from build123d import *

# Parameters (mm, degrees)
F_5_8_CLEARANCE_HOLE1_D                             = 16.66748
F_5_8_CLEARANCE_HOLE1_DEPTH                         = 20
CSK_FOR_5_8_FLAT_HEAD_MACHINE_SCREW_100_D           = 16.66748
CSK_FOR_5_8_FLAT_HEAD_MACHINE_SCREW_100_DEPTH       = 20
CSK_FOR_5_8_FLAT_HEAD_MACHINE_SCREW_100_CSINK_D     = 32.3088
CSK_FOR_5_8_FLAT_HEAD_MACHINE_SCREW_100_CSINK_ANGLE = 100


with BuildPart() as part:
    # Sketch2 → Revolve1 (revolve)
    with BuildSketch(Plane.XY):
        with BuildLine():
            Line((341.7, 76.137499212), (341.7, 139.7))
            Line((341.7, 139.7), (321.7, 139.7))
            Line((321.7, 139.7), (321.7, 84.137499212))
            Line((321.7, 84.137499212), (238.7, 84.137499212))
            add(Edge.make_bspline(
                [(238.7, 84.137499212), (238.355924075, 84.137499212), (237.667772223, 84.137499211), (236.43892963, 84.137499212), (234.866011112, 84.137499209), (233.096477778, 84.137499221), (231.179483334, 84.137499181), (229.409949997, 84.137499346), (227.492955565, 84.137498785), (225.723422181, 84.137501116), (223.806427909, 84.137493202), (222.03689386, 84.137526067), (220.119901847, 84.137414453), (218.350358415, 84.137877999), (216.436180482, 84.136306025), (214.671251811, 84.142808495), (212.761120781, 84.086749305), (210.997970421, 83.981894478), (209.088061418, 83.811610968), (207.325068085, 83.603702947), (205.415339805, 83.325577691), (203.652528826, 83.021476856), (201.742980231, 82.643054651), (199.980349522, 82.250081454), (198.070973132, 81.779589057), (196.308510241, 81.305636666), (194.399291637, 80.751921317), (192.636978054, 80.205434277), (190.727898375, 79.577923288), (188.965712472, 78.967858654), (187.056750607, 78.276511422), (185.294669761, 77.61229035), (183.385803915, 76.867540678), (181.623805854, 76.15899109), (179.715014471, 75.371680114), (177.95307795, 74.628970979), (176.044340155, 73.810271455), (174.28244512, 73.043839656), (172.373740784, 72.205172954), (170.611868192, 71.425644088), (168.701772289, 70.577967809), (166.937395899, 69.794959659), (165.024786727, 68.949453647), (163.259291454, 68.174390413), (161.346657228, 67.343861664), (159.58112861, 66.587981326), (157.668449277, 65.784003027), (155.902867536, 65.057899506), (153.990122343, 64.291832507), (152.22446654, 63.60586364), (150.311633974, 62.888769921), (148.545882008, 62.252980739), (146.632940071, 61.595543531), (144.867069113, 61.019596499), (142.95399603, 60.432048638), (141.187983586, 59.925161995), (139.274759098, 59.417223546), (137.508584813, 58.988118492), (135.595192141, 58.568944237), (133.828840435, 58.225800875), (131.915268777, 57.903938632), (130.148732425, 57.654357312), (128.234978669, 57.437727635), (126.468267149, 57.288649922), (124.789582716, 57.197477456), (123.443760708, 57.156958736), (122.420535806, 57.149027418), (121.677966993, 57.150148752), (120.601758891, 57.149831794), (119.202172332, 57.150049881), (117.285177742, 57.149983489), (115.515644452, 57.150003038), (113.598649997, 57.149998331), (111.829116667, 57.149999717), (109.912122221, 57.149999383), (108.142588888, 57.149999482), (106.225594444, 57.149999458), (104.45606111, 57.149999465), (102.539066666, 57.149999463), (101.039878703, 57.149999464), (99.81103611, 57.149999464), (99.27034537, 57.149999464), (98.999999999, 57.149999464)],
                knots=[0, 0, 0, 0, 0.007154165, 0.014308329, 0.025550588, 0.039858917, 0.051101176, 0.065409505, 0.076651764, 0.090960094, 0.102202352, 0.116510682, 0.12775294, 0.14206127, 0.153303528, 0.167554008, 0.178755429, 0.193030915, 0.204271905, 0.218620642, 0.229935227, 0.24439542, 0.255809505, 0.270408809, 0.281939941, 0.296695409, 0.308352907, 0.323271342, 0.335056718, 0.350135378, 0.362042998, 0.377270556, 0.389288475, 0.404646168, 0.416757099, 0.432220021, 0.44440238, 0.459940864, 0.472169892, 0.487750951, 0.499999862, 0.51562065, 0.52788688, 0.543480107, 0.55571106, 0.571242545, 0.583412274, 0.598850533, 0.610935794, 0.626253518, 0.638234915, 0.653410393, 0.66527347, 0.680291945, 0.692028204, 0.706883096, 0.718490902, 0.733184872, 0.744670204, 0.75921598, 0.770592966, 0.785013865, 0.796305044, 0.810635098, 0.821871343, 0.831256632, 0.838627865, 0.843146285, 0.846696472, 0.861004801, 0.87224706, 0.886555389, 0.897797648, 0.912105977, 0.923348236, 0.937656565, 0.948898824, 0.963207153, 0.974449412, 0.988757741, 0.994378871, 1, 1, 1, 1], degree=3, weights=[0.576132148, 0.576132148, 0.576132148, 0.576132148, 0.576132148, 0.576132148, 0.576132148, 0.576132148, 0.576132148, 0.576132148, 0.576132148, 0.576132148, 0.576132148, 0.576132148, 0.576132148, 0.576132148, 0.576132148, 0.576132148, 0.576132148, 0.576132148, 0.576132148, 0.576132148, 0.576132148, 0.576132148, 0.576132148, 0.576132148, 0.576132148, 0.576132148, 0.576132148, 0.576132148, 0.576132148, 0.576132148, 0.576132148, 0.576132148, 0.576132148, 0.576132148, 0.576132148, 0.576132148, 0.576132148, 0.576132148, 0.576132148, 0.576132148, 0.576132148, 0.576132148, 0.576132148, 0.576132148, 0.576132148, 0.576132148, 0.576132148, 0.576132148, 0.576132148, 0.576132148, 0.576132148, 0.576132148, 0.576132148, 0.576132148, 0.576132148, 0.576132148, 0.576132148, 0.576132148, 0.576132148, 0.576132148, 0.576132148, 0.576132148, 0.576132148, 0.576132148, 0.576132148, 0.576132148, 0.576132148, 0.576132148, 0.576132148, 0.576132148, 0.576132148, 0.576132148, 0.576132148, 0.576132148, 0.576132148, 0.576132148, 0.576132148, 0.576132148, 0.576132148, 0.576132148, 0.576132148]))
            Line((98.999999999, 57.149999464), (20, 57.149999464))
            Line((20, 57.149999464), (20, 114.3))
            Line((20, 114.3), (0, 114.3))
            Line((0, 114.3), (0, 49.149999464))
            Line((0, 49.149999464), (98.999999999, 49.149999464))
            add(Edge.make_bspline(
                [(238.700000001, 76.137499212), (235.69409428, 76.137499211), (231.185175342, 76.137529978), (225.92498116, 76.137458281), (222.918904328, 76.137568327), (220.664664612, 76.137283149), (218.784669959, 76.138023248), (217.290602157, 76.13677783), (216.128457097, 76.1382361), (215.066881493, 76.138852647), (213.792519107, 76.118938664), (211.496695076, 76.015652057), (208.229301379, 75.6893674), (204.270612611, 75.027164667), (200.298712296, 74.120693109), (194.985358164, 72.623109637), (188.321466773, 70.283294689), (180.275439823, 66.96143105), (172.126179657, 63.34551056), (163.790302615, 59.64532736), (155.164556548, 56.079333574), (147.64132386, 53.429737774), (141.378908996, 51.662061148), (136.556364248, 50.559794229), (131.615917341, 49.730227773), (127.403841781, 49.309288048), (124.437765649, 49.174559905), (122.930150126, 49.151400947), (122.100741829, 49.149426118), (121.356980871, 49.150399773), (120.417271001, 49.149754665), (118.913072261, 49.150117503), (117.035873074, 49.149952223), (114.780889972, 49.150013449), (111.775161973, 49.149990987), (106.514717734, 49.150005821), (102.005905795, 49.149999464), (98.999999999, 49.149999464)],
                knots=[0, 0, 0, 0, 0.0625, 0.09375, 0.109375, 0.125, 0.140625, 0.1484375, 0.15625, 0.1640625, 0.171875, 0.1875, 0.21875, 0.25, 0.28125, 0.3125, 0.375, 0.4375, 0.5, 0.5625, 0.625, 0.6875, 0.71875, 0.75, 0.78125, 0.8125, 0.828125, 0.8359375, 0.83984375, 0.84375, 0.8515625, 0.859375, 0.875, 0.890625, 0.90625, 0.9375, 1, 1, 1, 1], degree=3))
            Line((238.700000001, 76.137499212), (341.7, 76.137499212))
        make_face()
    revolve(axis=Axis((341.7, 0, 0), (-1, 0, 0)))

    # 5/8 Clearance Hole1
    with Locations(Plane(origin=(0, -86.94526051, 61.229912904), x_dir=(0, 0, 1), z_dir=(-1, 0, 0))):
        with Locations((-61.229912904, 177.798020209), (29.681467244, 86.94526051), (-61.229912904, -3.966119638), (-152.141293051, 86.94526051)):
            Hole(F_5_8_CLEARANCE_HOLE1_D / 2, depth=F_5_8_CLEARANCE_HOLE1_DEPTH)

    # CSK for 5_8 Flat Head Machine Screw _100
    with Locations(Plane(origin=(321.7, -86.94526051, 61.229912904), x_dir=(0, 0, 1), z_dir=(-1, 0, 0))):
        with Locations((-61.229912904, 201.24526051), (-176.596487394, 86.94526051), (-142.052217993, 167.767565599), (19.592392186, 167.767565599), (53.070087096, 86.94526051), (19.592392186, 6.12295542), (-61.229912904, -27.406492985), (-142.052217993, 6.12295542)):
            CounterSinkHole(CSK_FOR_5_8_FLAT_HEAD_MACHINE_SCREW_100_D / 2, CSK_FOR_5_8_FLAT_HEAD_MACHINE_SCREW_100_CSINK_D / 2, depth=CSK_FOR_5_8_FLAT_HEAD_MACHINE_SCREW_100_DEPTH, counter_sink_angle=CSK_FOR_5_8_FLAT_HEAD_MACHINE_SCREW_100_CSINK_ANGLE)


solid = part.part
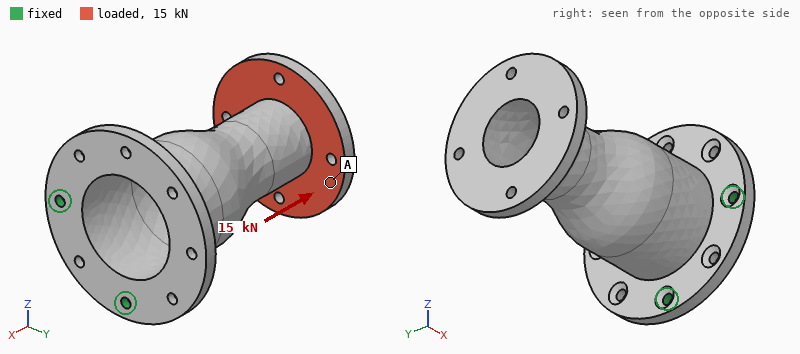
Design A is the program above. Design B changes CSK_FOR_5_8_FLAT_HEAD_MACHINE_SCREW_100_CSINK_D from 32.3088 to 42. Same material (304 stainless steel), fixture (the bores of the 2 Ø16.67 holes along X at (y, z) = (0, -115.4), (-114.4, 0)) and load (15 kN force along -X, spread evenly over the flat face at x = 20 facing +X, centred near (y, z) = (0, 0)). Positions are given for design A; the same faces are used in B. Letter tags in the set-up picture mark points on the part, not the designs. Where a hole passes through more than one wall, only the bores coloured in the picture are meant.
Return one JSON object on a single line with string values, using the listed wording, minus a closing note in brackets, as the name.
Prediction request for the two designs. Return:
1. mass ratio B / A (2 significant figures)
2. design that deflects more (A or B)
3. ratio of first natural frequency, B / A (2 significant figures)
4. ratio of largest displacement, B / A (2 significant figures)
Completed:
{"mass ratio B / A": "0.99", "design that deflects more": "B", "ratio of first natural frequency, B / A": "0.86", "ratio of largest displacement, B / A": "1.4"}
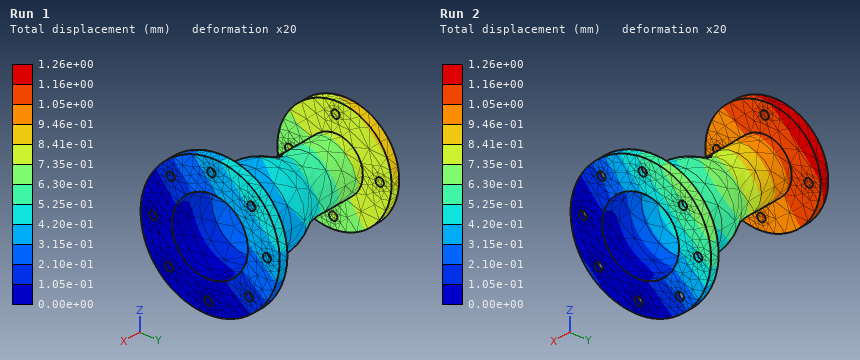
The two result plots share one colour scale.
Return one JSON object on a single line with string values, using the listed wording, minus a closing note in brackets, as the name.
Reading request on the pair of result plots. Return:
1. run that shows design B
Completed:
{"run that shows design B": "Run 2"}
